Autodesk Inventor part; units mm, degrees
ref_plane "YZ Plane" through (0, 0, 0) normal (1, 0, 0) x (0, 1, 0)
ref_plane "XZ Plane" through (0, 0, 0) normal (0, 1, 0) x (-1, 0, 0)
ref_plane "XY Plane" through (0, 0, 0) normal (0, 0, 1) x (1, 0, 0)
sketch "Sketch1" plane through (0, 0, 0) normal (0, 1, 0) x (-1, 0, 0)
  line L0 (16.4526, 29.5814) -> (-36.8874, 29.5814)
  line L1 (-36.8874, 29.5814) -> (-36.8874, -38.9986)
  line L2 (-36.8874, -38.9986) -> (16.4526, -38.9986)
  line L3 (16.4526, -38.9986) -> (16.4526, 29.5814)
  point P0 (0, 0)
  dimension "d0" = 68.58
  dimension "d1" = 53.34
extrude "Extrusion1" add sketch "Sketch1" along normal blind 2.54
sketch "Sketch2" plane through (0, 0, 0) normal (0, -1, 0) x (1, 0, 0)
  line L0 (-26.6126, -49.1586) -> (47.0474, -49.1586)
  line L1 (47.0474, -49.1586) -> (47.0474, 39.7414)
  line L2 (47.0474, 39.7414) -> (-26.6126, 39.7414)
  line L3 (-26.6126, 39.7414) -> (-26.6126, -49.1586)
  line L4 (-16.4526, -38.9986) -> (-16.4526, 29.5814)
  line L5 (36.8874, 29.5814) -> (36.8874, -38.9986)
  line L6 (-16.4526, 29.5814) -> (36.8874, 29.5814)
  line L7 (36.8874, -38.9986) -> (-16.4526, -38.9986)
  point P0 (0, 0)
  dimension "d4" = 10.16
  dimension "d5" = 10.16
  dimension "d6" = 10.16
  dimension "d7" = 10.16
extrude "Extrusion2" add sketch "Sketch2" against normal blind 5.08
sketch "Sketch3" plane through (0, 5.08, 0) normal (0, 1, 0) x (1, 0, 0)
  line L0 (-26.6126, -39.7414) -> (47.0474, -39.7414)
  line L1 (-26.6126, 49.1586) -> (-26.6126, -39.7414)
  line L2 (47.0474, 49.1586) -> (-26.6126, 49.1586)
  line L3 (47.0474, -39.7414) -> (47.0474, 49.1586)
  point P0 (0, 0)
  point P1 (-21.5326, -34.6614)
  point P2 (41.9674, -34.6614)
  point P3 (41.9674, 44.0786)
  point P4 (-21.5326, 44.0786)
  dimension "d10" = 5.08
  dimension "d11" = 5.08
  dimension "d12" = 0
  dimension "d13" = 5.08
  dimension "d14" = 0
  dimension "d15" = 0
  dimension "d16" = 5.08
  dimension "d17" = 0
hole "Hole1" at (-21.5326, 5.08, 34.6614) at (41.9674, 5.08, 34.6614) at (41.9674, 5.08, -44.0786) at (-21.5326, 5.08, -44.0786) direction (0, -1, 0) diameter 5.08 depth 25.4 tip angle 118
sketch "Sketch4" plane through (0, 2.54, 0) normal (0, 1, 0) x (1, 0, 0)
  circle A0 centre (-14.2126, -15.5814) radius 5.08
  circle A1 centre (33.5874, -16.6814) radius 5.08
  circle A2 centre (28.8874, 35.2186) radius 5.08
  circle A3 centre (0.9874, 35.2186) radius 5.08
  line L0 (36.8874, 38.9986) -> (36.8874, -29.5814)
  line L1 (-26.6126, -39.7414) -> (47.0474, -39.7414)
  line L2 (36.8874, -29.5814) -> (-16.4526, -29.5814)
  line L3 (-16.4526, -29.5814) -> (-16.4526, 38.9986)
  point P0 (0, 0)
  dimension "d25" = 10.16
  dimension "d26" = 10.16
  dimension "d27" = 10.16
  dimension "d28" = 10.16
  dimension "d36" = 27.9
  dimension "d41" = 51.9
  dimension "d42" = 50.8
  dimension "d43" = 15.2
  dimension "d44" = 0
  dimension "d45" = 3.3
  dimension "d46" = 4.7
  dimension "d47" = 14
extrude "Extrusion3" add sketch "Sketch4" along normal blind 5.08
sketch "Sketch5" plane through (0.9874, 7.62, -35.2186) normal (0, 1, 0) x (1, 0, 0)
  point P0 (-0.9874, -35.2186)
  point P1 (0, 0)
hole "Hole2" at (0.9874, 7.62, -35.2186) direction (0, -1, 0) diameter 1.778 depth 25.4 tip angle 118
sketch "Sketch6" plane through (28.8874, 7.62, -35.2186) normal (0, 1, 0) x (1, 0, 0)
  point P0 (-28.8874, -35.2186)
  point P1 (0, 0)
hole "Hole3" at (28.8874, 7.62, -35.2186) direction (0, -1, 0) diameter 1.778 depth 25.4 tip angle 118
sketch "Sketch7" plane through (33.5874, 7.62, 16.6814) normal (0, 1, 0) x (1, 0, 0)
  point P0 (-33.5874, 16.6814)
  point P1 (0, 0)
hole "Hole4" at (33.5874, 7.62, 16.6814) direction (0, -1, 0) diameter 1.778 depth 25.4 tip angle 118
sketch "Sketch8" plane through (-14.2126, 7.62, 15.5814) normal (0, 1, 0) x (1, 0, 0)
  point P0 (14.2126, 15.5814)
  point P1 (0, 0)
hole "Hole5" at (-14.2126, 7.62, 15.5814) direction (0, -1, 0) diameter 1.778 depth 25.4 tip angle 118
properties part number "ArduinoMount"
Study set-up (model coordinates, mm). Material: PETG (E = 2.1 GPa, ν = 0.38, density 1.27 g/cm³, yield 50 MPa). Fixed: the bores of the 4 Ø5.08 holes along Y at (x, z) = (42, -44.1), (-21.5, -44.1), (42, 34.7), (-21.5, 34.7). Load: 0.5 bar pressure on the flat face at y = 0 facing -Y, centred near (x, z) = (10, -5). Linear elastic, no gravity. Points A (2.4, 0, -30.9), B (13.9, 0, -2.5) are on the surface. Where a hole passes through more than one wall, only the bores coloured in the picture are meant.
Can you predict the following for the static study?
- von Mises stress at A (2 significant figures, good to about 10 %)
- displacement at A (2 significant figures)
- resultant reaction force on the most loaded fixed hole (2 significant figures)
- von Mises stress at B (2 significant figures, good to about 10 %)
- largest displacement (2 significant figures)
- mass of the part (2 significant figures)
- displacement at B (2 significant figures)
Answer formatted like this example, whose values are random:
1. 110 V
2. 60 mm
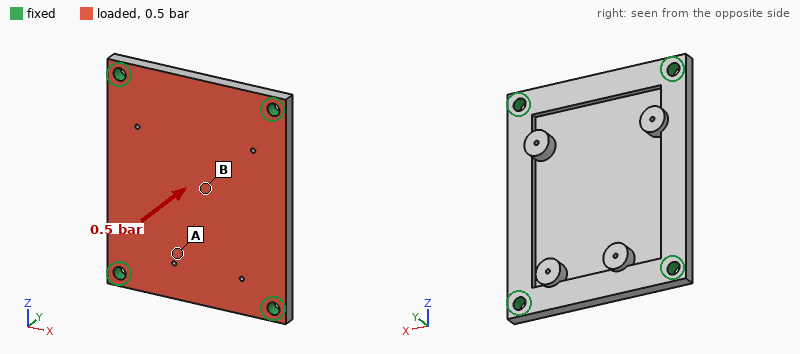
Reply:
1. 2.2 MPa
2. 0.40 mm
3. 110 N
4. 7.3 MPa
5. 0.87 mm
6. 32 g
7. 0.86 mm
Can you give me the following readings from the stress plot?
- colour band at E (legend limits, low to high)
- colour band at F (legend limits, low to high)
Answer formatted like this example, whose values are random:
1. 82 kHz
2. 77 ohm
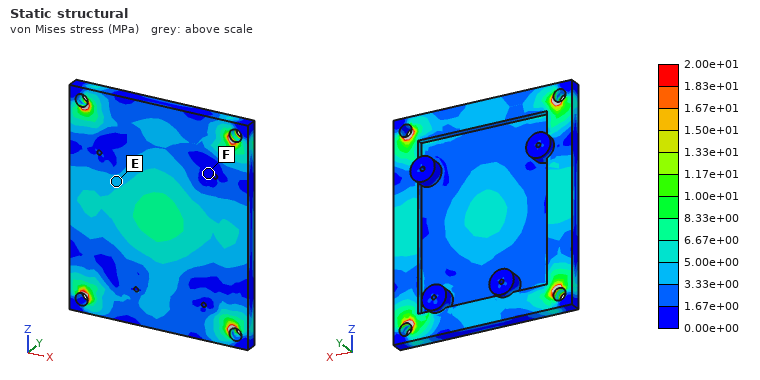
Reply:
1. 3.33e+00 to 5.00e+00 MPa
2. 0.00e+00 to 1.67e+00 MPa
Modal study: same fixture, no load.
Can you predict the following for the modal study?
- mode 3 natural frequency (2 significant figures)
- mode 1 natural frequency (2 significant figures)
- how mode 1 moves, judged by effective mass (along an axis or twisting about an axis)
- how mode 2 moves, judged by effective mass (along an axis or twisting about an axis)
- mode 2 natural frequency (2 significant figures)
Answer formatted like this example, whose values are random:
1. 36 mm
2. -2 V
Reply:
1. 1400 Hz
2. 800 Hz
3. along Y
4. twisting about Z
5. 1100 Hz
